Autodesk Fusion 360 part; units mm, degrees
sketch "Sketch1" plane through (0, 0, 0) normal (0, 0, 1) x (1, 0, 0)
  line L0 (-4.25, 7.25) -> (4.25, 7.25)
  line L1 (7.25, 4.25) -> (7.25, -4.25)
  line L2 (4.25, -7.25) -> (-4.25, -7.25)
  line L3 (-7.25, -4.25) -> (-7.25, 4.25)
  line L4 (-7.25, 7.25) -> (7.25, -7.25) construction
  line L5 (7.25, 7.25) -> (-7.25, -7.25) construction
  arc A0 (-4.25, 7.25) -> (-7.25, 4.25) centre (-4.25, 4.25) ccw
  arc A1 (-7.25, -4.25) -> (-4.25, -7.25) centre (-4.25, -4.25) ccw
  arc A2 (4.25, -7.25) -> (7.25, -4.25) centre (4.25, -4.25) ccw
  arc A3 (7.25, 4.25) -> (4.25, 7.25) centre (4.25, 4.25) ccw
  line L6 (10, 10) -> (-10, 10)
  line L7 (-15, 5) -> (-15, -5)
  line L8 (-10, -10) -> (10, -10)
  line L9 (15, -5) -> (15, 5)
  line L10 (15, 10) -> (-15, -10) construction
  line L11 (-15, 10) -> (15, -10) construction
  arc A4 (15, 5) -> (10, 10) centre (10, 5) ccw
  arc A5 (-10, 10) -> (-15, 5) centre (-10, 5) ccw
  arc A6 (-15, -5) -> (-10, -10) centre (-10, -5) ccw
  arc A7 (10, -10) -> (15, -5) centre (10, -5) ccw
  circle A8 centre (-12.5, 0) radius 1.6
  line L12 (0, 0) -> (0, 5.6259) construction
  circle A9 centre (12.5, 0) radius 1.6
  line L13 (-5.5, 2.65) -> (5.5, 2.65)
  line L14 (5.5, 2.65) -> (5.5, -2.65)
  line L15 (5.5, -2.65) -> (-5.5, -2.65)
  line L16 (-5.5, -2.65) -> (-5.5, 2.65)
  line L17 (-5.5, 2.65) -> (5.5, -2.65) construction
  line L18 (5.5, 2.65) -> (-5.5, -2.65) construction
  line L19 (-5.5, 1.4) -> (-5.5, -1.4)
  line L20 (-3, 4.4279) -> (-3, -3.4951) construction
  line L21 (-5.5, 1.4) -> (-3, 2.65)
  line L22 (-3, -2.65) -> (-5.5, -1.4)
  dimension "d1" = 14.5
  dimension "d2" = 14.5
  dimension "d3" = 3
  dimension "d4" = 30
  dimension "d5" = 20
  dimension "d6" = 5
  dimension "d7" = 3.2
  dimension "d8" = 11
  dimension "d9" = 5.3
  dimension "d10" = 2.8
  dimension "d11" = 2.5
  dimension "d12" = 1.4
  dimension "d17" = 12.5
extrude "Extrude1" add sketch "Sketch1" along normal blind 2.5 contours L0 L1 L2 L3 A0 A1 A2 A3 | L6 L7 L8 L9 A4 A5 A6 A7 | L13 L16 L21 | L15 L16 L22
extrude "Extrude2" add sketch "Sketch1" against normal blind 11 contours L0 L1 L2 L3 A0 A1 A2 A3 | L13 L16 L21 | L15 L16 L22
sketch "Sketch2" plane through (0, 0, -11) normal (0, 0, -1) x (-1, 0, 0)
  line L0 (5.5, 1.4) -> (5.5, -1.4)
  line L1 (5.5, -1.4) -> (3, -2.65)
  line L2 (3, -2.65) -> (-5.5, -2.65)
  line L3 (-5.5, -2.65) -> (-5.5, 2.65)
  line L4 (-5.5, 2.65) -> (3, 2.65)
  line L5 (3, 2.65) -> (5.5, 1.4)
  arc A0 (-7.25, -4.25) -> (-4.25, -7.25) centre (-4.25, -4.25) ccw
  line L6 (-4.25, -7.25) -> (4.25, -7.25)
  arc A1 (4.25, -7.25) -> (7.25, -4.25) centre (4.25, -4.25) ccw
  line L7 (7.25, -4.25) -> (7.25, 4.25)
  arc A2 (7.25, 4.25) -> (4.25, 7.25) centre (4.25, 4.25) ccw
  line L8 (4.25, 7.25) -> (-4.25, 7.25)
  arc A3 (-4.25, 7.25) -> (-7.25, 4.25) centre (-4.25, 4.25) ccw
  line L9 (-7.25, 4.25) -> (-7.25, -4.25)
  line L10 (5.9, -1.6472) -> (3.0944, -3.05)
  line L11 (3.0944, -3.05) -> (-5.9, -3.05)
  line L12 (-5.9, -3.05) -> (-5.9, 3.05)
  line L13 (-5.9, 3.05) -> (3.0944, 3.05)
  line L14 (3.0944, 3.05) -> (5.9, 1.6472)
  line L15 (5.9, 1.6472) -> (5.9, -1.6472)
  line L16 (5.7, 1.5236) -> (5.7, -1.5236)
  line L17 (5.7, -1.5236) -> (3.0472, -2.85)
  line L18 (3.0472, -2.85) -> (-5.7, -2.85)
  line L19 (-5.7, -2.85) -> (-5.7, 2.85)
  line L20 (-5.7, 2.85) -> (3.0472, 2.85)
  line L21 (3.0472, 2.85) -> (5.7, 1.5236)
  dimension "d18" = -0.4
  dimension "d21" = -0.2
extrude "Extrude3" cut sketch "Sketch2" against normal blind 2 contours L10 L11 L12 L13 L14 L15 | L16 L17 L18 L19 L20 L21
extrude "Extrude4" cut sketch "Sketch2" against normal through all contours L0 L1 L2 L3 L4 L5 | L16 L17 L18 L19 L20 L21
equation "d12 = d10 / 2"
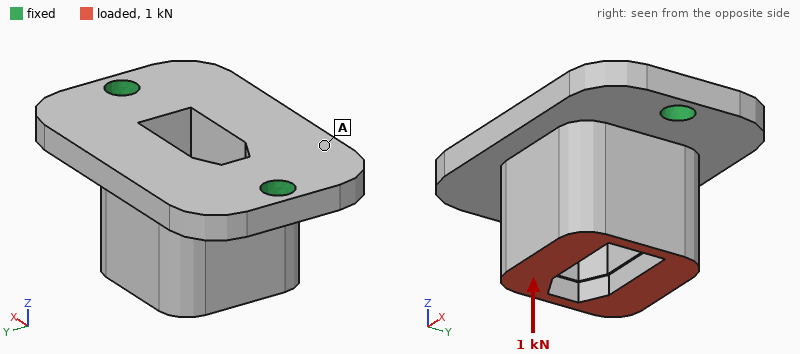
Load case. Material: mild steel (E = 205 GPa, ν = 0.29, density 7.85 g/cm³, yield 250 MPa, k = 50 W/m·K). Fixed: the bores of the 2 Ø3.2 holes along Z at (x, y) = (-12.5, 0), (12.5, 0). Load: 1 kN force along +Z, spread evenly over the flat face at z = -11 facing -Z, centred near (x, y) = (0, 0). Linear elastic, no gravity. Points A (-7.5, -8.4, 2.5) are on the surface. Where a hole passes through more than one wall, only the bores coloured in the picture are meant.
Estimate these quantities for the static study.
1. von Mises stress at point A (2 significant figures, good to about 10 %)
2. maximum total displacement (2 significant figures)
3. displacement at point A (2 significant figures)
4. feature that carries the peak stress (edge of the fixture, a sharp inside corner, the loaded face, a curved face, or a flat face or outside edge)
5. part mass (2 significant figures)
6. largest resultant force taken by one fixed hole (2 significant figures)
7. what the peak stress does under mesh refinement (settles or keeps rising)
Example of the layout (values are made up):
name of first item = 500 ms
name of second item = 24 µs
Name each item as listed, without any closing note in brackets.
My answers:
von Mises stress at point A = 23 MPa
maximum total displacement = 5.9 µm
displacement at point A = 4.6 µm
feature that carries the peak stress = edge of the fixture
part mass = 22 g
largest resultant force taken by one fixed hole = 540 N
what the peak stress does under mesh refinement = keeps rising
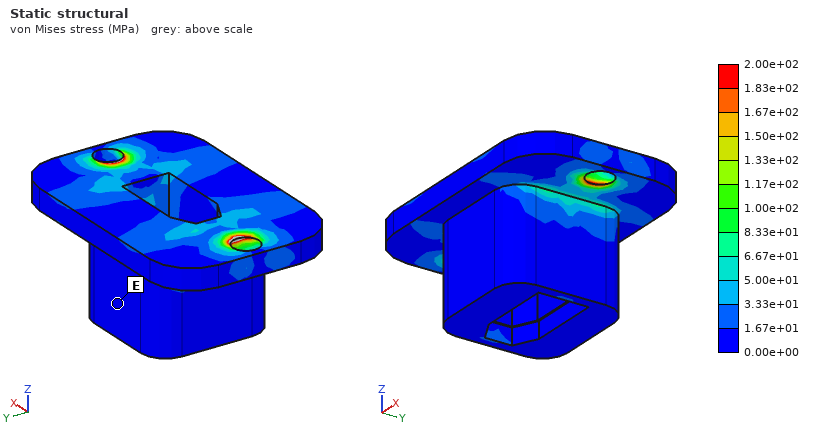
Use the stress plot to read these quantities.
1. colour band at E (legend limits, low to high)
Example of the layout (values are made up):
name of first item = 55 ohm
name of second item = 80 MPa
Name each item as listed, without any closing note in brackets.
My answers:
colour band at E = 0.00e+00 to 1.67e+01 MPa
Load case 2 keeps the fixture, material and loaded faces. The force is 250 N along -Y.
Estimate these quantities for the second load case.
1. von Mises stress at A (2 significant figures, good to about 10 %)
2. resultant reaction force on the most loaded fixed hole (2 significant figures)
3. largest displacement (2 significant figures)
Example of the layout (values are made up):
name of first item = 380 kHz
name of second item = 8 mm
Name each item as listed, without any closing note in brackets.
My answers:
von Mises stress at A = 25 MPa
resultant reaction force on the most loaded fixed hole = 130 N
largest displacement = 18 µm
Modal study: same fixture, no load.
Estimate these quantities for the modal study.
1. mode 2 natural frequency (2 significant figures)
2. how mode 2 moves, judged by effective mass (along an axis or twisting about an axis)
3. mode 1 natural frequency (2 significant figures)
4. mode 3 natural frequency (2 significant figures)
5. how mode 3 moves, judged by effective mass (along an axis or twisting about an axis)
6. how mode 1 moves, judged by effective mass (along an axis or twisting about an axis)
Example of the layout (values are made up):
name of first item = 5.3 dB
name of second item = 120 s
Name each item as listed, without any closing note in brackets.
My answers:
mode 2 natural frequency = 16 kHz
how mode 2 moves, judged by effective mass = along Z
mode 1 natural frequency = 7300 Hz
mode 3 natural frequency = 20 kHz
how mode 3 moves, judged by effective mass = along X
how mode 1 moves, judged by effective mass = along Y
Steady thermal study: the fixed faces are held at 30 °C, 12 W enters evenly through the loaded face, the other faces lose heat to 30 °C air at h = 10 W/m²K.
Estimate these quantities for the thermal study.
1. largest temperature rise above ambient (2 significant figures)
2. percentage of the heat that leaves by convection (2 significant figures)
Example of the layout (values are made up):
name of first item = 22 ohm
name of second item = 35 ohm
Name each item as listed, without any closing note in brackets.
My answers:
largest temperature rise above ambient = 43 K
percentage of the heat that leaves by convection = 4.1 %
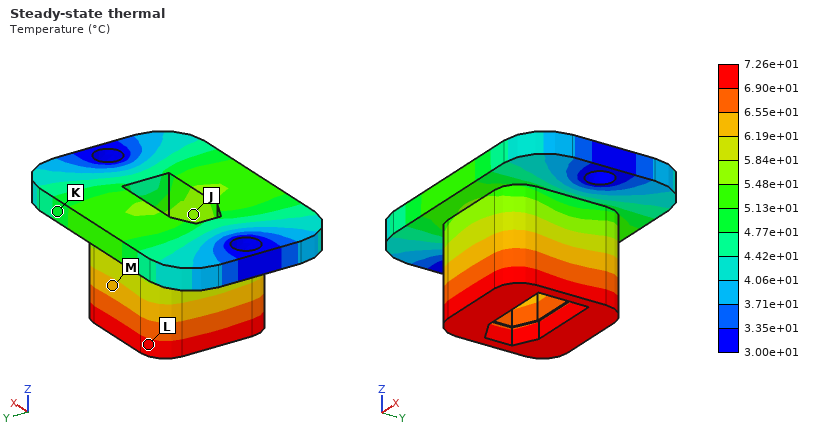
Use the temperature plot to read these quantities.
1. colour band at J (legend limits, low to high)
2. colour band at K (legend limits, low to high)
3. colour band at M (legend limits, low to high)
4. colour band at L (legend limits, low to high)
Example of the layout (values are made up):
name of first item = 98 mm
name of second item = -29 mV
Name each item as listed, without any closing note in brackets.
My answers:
colour band at J = 5.48e+01 to 5.84e+01 °C
colour band at K = 4.77e+01 to 5.13e+01 °C
colour band at M = 6.19e+01 to 6.55e+01 °C
colour band at L = 6.90e+01 to 7.26e+01 °C
